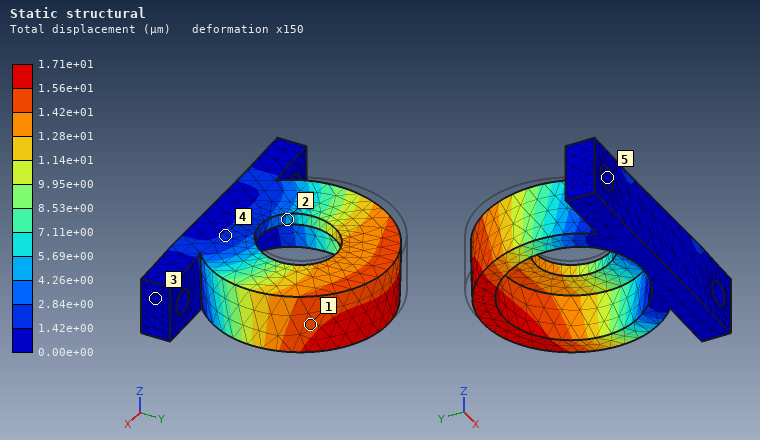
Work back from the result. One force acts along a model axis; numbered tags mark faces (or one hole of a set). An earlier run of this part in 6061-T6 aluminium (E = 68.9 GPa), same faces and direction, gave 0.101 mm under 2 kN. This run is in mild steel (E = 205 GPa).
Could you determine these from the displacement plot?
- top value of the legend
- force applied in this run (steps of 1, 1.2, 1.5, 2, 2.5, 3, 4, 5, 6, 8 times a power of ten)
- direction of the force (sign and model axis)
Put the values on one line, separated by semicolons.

1.71e+01 µm; 1 kN; +X
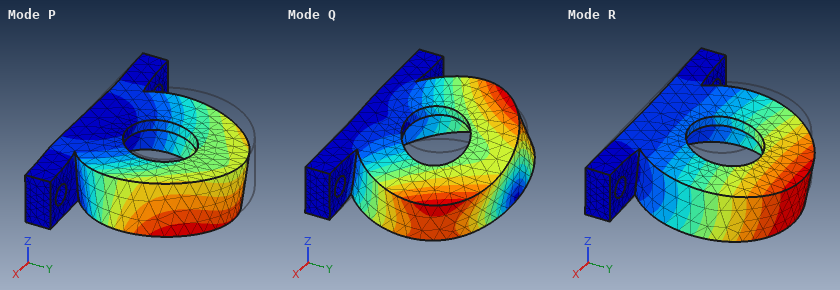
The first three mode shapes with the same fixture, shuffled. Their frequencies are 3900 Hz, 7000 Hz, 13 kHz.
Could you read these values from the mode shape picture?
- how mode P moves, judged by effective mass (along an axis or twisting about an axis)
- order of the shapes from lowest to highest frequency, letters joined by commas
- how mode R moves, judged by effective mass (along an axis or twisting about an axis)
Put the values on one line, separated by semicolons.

along X; R, P, Q; along Z
